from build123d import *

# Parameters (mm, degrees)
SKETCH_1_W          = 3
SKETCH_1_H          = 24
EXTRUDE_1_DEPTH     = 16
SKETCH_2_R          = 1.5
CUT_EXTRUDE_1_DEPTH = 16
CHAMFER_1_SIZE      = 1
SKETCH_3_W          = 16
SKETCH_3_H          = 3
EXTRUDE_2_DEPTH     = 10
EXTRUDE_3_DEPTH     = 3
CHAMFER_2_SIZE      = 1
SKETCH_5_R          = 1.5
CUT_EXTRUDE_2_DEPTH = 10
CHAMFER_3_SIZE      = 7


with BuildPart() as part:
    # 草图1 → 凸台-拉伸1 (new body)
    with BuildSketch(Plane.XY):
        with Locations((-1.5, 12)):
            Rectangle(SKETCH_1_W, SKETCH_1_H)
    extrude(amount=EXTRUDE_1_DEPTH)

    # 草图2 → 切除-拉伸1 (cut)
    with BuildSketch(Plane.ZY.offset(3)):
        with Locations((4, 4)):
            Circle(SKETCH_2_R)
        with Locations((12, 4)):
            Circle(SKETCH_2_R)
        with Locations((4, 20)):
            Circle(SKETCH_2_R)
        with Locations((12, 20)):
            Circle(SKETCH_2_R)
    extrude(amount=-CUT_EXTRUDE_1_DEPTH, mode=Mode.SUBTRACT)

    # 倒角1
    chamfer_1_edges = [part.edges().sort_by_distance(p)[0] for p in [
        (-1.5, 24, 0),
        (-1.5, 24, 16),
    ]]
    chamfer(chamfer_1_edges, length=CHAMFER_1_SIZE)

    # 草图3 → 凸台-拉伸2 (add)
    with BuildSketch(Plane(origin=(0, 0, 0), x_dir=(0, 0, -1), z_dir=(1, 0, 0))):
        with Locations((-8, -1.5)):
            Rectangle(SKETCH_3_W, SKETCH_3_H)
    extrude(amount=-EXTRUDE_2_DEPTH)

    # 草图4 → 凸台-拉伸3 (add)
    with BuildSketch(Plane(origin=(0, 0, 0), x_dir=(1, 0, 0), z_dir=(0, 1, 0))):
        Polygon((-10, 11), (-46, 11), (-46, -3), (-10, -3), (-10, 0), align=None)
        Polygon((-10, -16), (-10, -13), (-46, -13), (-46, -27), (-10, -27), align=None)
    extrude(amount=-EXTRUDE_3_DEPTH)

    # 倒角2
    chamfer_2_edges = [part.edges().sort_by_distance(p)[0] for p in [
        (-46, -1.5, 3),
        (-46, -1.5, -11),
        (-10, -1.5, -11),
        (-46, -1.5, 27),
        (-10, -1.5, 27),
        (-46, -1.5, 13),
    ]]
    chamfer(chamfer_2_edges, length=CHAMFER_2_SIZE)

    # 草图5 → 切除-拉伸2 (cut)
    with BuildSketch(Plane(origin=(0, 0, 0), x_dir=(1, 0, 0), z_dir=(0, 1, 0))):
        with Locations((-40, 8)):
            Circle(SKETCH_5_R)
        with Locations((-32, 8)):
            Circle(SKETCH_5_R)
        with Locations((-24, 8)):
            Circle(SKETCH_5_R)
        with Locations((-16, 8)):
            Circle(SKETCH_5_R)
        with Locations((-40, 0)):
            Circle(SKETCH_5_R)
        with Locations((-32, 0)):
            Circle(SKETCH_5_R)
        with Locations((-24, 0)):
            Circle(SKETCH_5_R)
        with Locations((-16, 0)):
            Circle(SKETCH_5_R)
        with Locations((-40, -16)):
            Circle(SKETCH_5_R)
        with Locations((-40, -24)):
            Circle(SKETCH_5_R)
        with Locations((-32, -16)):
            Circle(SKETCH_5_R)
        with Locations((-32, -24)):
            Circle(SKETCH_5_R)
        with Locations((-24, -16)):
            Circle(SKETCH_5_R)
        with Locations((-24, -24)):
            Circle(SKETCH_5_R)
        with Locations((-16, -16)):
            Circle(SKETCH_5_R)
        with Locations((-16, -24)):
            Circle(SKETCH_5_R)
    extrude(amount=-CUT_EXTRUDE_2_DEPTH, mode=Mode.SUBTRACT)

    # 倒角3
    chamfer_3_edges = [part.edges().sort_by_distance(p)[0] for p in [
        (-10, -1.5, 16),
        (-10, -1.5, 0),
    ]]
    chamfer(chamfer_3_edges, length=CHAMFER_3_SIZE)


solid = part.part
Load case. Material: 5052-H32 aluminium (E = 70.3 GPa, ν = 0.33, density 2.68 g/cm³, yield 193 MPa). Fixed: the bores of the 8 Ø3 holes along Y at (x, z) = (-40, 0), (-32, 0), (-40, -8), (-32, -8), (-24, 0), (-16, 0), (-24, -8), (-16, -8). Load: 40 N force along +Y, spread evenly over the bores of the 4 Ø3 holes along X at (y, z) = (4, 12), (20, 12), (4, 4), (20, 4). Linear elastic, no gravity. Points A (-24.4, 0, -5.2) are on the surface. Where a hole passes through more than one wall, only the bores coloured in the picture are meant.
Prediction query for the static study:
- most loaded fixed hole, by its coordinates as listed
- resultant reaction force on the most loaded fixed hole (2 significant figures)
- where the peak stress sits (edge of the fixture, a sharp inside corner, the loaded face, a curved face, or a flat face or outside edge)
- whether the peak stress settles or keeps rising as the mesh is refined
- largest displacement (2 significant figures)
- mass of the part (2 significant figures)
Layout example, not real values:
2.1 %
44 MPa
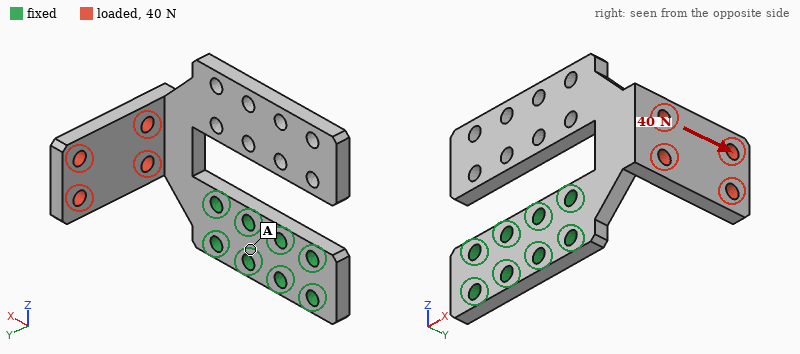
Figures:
(-16, 0)
69 N
edge of the fixture
keeps rising
0.11 mm
12 g
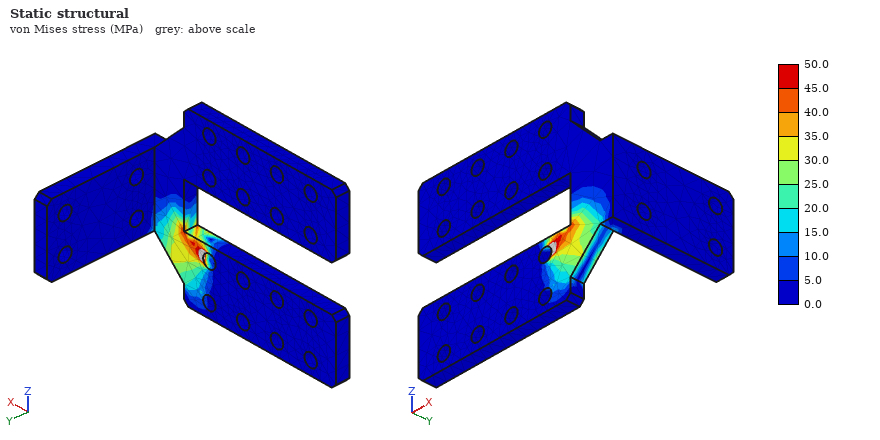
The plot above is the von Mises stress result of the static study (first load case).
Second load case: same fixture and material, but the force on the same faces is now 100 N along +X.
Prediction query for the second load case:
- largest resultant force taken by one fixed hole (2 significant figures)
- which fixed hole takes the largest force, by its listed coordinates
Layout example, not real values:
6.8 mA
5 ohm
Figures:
180 N
(-16, 0)
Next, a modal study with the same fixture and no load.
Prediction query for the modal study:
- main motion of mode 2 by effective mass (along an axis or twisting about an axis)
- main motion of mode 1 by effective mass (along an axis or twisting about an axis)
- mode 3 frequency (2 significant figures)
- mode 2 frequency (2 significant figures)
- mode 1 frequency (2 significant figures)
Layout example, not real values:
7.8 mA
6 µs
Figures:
along Y
along Y
1900 Hz
1400 Hz
740 Hz
